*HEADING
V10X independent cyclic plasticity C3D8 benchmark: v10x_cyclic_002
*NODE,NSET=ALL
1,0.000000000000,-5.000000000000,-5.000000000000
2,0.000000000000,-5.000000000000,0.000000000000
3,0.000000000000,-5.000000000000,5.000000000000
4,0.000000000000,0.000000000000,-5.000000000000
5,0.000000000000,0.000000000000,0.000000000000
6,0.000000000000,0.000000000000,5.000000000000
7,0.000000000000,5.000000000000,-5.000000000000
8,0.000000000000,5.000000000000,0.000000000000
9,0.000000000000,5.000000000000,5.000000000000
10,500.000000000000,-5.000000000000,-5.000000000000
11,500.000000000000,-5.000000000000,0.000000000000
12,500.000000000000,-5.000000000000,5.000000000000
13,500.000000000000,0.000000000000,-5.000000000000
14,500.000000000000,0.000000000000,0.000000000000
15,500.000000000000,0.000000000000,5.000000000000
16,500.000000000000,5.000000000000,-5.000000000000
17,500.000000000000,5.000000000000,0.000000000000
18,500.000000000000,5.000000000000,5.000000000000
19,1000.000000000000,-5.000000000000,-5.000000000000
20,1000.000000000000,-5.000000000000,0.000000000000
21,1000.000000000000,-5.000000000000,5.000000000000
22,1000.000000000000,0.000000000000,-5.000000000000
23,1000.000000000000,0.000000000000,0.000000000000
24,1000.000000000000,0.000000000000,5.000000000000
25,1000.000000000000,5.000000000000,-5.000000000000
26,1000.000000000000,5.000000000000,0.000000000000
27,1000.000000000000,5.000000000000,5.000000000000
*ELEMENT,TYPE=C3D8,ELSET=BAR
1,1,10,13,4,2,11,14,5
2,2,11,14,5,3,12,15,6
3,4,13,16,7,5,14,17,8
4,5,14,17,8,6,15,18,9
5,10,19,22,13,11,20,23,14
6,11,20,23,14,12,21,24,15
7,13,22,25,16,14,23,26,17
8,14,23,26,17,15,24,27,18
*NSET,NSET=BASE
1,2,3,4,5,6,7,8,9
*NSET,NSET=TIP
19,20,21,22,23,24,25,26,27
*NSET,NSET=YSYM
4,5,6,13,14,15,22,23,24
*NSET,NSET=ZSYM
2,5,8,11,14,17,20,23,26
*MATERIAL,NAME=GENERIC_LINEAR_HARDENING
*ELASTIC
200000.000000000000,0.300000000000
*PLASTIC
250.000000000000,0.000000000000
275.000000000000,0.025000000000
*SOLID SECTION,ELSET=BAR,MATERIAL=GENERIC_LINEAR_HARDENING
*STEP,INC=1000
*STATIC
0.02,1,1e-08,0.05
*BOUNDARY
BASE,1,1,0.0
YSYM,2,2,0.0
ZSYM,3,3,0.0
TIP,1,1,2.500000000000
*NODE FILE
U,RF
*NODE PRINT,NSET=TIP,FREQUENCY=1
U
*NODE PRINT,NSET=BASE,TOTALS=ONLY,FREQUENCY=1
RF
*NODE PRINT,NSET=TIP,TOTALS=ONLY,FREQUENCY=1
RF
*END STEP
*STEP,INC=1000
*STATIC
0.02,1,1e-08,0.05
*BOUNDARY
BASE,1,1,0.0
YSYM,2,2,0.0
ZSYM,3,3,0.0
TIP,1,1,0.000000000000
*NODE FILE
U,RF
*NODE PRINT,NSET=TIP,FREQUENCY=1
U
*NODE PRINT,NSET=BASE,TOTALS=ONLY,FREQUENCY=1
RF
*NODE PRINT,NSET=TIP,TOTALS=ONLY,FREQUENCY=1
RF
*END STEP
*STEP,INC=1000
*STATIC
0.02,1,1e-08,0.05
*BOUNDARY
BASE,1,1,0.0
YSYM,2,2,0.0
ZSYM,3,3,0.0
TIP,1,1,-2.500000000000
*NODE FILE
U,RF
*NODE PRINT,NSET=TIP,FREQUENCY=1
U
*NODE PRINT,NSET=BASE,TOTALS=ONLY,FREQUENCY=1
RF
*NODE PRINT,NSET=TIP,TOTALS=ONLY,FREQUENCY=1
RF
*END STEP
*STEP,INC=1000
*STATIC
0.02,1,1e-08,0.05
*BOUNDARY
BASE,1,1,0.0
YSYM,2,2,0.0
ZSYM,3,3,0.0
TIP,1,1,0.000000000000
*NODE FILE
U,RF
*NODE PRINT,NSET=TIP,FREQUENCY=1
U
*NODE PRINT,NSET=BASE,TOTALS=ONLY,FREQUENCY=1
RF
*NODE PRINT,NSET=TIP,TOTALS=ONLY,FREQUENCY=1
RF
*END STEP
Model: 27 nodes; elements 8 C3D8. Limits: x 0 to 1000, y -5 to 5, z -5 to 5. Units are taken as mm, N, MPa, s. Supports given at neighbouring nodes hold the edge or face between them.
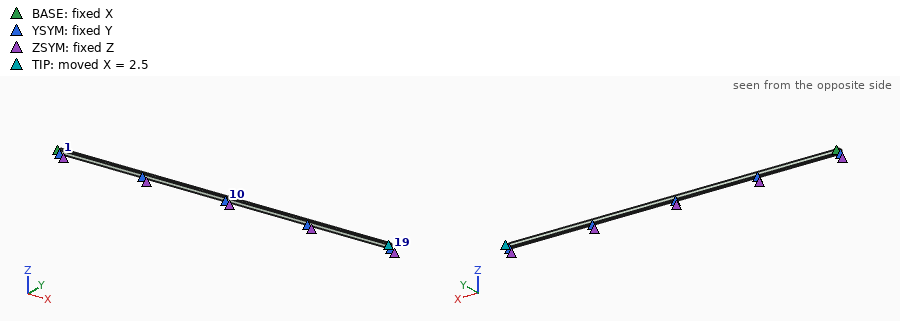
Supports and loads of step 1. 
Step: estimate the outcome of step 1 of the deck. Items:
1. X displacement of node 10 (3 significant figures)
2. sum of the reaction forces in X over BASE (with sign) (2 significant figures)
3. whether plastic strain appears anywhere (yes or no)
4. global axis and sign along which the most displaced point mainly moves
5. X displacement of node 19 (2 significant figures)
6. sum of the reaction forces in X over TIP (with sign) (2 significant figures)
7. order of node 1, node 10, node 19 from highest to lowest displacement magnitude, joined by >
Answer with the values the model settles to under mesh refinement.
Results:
1.25 mm
-25000 N
yes
+X
2.5 mm
25000 N
node 19 > node 10 > node 1
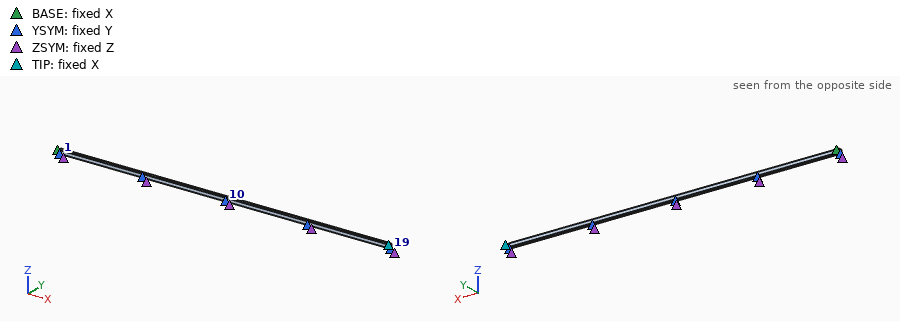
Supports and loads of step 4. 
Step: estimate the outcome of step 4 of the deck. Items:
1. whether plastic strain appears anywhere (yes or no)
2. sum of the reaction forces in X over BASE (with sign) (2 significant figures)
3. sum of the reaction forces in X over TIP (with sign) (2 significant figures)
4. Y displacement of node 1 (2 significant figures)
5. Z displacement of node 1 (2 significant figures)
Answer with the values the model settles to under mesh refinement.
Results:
yes
-25000 N
25000 N
-0.0012 mm
-0.0012 mm
